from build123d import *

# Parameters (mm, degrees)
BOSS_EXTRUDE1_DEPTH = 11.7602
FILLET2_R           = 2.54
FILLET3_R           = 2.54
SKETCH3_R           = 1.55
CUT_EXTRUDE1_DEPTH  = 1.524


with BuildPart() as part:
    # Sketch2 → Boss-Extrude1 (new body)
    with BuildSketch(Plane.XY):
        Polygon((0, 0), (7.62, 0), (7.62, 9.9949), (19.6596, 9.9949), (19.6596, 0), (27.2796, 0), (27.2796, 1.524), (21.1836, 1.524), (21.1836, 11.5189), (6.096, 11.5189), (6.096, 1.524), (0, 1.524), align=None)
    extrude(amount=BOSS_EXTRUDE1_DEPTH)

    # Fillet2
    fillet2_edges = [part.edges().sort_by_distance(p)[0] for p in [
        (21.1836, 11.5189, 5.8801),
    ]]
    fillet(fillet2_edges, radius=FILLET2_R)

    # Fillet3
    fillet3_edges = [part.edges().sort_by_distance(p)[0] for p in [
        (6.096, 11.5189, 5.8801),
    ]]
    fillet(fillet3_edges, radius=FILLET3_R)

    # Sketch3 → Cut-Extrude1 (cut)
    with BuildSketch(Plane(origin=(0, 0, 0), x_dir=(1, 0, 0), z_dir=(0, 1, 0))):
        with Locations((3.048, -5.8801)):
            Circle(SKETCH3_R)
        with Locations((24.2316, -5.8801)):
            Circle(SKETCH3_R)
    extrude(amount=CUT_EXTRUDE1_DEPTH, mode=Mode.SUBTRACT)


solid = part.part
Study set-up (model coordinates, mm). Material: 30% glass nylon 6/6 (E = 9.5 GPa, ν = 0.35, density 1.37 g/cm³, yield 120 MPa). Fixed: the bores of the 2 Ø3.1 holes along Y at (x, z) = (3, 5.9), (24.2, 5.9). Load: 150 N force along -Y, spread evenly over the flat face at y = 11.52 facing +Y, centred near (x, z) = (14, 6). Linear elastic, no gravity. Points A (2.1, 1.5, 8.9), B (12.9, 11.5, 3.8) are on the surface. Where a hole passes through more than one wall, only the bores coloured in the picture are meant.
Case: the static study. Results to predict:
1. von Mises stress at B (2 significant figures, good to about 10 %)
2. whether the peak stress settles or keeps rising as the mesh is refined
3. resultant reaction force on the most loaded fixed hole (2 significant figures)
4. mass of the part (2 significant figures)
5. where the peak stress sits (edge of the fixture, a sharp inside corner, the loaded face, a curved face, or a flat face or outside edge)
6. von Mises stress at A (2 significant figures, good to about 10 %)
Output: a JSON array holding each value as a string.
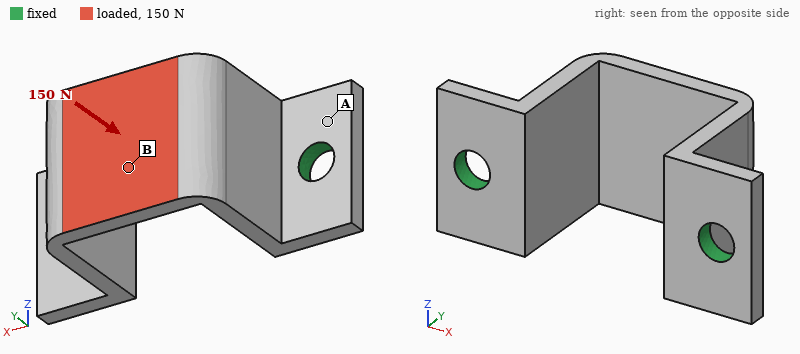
["32 MPa", "keeps rising", "80 N", "1.1 g", "edge of the fixture", "5.0 MPa"]
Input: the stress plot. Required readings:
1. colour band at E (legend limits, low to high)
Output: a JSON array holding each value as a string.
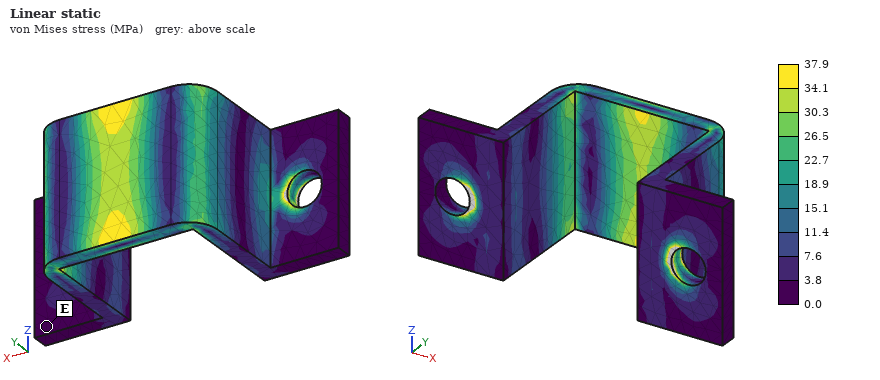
["0.0 to 3.8 MPa"]
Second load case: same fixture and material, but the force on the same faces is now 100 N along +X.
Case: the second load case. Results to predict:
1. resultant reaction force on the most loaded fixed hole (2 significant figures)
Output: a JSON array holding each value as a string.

["65 N"]
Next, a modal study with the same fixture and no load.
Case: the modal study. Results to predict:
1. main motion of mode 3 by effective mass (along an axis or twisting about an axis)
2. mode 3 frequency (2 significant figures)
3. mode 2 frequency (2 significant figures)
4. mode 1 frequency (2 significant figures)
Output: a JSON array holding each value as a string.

["twisting about Y", "7000 Hz", "4600 Hz", "4500 Hz"]
